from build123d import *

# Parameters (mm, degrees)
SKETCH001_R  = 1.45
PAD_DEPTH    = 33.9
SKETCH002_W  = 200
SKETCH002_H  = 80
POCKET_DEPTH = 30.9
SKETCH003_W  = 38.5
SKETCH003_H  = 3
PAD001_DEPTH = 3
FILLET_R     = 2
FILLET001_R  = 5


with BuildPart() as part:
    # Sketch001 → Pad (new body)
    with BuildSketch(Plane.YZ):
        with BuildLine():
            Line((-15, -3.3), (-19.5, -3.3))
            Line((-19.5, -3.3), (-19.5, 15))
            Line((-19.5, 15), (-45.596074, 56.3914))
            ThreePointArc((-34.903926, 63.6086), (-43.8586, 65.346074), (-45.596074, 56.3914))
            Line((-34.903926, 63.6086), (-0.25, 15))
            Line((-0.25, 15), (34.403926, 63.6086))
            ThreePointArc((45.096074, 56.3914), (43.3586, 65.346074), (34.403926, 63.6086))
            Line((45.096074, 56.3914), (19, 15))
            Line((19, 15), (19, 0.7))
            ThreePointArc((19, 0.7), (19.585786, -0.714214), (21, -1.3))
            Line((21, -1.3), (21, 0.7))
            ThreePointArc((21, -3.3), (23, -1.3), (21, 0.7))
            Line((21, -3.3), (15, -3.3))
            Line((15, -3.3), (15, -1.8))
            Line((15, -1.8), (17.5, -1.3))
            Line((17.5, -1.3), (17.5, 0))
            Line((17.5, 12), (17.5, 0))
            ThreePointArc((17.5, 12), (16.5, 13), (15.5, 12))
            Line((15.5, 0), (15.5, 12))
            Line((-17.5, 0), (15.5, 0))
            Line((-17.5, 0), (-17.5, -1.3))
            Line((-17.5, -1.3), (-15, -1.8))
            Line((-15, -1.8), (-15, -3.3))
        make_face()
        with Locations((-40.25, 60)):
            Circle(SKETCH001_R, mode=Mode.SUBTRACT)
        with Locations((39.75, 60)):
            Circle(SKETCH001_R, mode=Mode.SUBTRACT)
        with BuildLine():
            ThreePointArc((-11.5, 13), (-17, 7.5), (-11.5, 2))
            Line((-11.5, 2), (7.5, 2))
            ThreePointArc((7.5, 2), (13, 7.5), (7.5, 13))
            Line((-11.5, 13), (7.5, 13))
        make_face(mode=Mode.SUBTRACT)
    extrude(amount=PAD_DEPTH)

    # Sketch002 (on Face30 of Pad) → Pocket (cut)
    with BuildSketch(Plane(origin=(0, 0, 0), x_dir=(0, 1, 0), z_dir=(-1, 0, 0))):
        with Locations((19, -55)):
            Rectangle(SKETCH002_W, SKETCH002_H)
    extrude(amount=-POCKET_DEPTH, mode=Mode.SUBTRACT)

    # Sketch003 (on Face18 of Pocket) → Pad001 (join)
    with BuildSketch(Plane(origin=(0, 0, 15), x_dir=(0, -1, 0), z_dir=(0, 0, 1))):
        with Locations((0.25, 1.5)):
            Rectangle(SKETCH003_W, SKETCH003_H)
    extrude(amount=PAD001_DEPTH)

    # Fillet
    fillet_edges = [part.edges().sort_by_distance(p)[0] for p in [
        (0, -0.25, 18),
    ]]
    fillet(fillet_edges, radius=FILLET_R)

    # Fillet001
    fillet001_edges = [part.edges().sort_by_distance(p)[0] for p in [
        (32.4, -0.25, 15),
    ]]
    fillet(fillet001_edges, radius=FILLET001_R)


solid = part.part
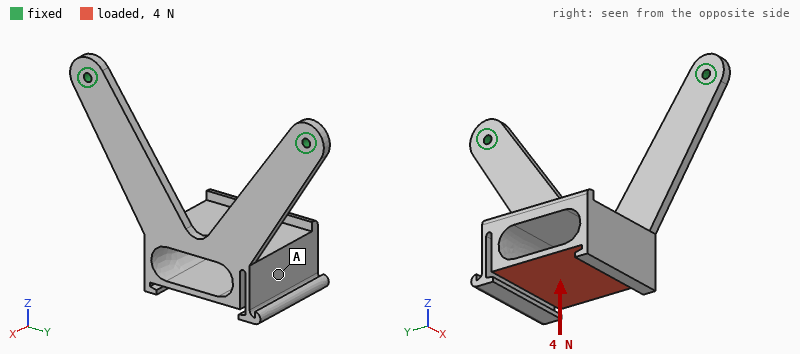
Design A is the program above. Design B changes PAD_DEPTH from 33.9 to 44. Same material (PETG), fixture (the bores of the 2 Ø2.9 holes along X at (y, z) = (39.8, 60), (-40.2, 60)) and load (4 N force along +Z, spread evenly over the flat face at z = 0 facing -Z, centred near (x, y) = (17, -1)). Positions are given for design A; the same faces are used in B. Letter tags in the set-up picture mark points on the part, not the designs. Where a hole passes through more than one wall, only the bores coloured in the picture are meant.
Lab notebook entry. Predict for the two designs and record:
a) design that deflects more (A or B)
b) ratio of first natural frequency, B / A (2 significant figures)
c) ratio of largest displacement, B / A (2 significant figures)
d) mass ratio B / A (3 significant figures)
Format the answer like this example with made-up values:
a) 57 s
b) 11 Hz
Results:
a) A
b) 6.3
c) 0.022
d) 2.34
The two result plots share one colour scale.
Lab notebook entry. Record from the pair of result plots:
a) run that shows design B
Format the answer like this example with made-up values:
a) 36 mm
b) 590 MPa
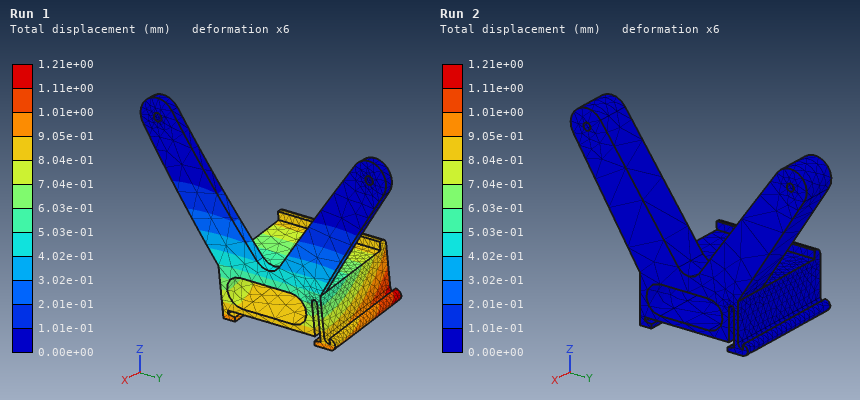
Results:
a) Run 2
